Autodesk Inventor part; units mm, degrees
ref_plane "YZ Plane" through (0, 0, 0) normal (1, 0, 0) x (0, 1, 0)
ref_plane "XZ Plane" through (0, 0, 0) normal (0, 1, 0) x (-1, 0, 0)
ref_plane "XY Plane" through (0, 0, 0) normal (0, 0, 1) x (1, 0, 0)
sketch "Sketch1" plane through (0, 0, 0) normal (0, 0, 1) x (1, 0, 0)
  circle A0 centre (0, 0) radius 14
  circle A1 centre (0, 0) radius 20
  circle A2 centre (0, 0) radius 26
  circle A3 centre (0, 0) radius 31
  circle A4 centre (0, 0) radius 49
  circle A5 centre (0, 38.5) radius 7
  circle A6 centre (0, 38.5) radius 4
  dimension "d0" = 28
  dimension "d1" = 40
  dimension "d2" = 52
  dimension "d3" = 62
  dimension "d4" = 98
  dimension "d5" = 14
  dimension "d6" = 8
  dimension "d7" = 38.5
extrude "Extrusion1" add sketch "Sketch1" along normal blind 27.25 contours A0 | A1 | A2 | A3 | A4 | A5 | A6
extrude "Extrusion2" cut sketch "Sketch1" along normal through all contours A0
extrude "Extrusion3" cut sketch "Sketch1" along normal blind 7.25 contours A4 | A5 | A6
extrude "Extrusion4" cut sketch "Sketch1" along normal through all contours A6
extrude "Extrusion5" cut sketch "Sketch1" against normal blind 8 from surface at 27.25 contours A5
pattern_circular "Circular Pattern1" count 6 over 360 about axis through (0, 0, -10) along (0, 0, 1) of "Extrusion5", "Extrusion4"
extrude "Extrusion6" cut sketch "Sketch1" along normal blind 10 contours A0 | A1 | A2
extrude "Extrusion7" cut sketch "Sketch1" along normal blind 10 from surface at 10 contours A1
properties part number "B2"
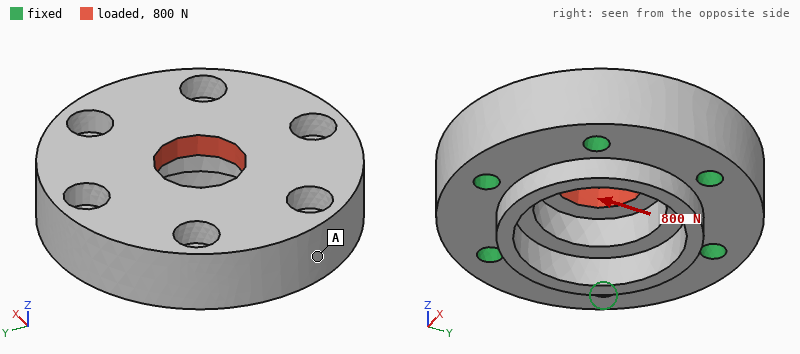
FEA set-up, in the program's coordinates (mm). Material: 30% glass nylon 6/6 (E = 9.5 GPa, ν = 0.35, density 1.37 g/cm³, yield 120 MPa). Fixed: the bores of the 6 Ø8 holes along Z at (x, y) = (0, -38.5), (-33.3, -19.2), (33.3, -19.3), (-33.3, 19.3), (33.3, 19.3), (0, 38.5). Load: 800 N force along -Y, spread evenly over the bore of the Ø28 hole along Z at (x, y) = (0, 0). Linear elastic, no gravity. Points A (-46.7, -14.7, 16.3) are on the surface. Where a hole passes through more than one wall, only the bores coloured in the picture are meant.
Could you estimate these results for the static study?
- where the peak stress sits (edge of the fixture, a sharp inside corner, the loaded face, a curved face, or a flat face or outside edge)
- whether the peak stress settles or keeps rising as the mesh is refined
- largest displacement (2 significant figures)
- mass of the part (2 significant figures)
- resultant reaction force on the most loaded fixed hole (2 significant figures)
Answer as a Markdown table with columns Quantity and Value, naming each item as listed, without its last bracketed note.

| Quantity | Value |
|---|---|
| where the peak stress sits | edge of the fixture |
| whether the peak stress settles or keeps rising as the mesh is refined | keeps rising |
| largest displacement | 5.0 µm |
| mass of the part | 170 g |
| resultant reaction force on the most loaded fixed hole | 190 N |
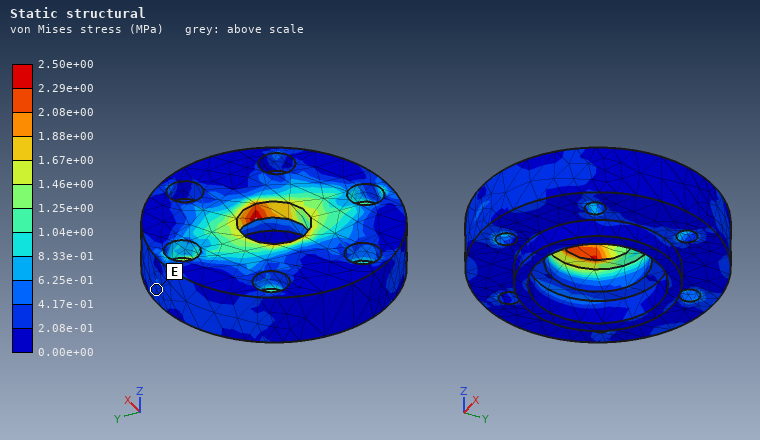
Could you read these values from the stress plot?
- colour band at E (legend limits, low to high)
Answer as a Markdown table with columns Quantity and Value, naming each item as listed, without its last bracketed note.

| Quantity | Value |
|---|---|
| colour band at E | 2.08e-01 to 4.17e-01 MPa |
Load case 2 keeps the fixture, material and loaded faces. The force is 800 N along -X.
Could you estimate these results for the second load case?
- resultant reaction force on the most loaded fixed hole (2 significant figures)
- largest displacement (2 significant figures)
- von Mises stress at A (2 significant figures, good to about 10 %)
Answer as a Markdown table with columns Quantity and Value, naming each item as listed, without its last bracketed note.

| Quantity | Value |
|---|---|
| resultant reaction force on the most loaded fixed hole | 170 N |
| largest displacement | 5.1 µm |
| von Mises stress at A | 0.36 MPa |
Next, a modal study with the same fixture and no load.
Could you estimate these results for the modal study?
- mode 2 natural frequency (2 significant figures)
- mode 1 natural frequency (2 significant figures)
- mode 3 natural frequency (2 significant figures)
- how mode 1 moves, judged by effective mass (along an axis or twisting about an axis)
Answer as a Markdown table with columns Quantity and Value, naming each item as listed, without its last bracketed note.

| Quantity | Value |
|---|---|
| mode 2 natural frequency | 12 kHz |
| mode 1 natural frequency | 11 kHz |
| mode 3 natural frequency | 12 kHz |
| how mode 1 moves, judged by effective mass | along Z |
